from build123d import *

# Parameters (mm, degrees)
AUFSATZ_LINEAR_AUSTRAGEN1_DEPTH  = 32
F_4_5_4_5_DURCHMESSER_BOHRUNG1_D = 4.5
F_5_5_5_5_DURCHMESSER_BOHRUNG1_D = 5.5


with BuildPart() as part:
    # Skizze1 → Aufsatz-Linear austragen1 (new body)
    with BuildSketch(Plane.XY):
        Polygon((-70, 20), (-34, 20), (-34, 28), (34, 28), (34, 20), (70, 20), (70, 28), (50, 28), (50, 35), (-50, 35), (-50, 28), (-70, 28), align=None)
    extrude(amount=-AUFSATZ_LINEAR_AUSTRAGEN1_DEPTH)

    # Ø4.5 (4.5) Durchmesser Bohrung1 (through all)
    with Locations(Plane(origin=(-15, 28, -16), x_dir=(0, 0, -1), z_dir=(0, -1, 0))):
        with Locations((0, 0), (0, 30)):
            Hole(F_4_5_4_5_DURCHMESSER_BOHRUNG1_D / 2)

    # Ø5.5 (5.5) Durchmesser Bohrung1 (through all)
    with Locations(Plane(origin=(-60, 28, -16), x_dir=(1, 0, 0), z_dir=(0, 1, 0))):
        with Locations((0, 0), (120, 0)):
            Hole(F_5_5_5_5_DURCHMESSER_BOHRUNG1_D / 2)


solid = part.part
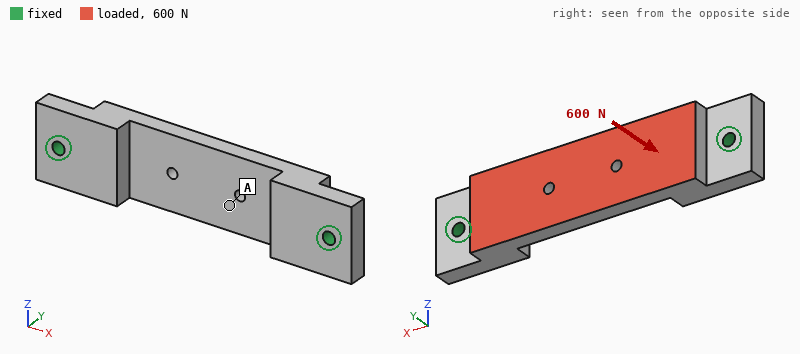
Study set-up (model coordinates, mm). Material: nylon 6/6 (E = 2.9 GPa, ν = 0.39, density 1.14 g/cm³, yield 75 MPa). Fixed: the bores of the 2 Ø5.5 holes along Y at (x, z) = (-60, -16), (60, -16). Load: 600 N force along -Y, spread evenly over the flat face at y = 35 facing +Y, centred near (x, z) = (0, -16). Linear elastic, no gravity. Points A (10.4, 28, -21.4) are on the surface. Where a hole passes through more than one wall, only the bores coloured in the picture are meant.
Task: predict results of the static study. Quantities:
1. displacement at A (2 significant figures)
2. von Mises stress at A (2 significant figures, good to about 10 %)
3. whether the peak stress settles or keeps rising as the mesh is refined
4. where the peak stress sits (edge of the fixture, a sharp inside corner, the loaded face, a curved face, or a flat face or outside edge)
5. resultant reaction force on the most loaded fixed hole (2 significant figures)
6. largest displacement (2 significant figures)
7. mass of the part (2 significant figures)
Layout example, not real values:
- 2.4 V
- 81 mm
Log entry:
- 0.46 mm
- 2.8 MPa
- keeps rising
- edge of the fixture
- 700 N
- 0.52 mm
- 46 g
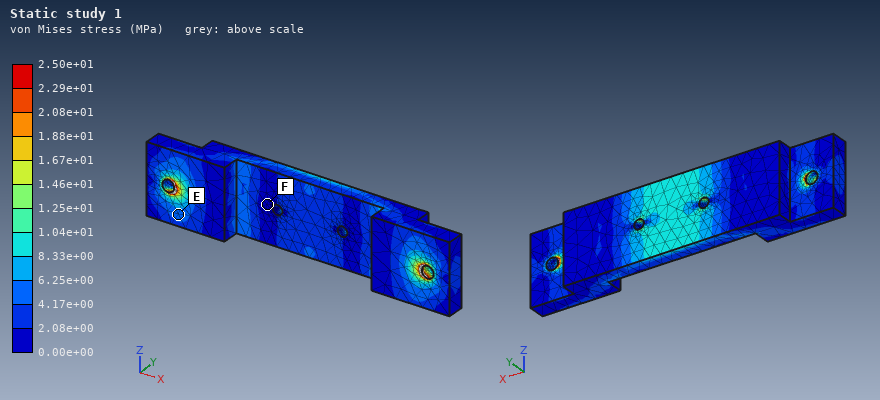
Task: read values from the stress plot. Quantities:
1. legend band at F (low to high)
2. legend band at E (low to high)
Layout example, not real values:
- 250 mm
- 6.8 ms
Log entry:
- 0.00e+00 to 2.08e+00 MPa
- 4.17e+00 to 6.25e+00 MPa
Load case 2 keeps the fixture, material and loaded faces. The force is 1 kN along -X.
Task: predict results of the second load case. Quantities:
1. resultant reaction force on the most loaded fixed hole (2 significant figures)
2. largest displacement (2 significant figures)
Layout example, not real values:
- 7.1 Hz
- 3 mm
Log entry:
- 510 N
- 0.12 mm
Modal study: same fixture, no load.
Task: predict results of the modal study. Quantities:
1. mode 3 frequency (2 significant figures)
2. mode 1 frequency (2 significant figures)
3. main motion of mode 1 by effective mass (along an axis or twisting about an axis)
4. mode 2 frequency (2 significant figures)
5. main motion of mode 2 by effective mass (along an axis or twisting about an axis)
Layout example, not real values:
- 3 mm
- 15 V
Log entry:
- 1800 Hz
- 1200 Hz
- along Y
- 1500 Hz
- along Z
